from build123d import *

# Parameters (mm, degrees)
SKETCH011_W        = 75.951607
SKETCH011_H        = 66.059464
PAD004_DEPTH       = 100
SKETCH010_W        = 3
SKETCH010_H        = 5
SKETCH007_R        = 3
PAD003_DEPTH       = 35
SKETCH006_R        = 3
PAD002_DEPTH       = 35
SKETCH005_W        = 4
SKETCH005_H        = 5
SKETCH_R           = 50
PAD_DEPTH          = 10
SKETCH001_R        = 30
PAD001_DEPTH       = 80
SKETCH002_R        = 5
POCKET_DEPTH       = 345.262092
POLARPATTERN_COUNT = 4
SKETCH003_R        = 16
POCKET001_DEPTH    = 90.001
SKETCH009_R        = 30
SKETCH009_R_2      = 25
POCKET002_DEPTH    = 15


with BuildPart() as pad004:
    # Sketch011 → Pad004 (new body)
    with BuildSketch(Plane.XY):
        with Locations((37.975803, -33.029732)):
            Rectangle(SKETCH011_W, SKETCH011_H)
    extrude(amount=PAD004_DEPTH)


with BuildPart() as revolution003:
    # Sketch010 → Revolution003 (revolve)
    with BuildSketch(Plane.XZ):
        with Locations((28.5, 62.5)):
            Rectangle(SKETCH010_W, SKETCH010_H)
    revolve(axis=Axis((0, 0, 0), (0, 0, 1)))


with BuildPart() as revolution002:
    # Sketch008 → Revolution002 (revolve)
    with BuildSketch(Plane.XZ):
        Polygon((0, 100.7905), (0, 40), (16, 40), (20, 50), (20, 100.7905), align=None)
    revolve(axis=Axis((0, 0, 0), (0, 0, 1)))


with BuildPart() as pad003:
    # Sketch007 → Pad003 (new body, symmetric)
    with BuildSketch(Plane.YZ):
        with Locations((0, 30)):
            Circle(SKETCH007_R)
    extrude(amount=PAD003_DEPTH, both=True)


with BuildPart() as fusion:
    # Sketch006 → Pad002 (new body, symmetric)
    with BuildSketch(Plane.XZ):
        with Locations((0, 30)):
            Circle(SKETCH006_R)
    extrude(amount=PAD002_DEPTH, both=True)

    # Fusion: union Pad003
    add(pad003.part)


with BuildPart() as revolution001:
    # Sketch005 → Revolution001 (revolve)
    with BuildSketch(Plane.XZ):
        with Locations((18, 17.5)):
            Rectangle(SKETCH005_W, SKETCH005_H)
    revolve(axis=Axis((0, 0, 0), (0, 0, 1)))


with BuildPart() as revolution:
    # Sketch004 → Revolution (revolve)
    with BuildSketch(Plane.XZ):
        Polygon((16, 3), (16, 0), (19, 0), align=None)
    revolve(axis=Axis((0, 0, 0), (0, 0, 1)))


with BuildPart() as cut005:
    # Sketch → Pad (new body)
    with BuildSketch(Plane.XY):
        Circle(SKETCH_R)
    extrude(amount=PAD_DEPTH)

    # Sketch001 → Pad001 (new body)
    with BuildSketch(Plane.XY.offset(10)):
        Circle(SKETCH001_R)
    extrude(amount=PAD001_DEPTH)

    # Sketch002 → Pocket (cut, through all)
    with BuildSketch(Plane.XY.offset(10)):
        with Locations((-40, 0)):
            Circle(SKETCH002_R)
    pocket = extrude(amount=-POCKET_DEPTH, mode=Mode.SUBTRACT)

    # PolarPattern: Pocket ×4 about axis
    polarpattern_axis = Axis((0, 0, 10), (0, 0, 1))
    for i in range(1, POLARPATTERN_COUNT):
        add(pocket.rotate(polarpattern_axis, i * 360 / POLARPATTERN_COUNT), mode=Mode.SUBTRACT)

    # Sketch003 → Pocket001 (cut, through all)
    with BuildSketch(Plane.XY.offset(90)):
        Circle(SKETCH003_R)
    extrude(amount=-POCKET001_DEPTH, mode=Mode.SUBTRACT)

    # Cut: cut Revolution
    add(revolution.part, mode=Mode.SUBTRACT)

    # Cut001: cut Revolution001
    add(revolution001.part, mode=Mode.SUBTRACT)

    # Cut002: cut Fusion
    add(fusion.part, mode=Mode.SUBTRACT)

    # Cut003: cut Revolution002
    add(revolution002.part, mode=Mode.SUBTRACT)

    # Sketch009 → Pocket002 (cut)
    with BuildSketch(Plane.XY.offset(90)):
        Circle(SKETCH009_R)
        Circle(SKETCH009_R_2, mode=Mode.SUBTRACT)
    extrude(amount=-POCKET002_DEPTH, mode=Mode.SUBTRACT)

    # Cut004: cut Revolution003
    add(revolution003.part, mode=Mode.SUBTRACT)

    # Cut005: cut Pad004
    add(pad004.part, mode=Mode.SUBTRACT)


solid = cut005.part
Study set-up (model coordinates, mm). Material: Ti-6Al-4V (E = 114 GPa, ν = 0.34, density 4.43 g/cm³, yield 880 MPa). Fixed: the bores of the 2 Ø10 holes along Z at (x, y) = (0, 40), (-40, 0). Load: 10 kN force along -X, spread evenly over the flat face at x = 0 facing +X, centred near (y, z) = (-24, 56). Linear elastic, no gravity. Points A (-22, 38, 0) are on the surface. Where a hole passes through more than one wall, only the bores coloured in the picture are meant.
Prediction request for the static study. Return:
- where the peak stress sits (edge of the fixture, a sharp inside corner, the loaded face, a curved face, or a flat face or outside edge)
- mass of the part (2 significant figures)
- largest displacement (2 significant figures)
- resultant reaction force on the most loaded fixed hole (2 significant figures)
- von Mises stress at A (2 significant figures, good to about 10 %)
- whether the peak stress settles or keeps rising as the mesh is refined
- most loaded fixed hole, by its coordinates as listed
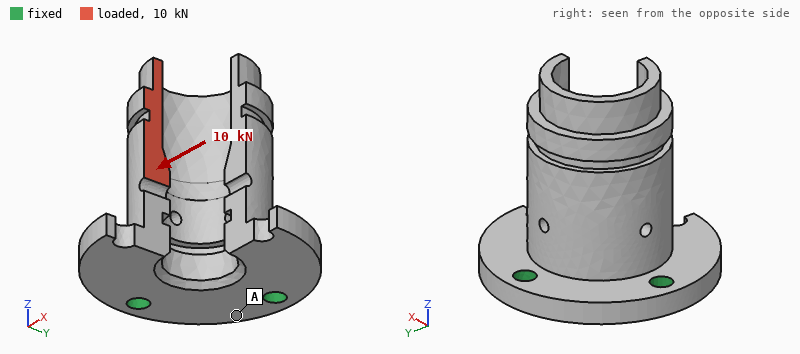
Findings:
edge of the fixture
630 g
0.98 mm
12 kN
43 MPa
keeps rising
(-40, 0)
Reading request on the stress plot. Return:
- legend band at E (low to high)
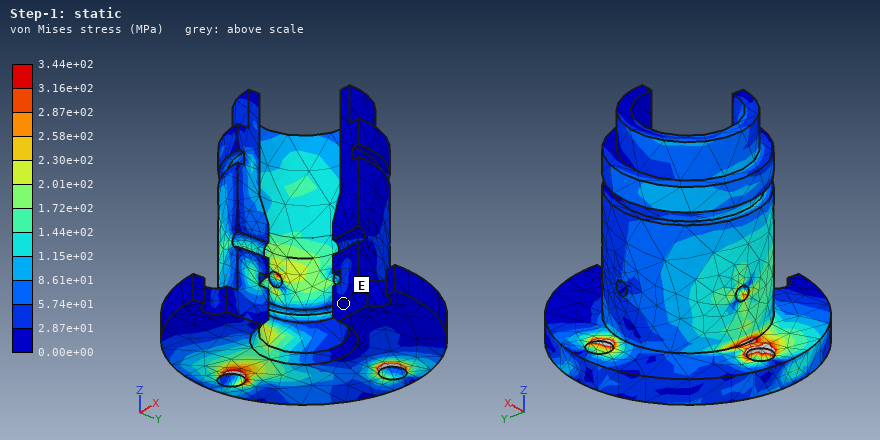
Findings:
0.00e+00 to 2.87e+01 MPa
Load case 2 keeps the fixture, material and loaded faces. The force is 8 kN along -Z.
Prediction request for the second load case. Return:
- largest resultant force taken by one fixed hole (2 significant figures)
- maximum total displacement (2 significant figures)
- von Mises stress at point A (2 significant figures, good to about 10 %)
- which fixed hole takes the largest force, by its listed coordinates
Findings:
7.0 kN
0.59 mm
45 MPa
(-40, 0)
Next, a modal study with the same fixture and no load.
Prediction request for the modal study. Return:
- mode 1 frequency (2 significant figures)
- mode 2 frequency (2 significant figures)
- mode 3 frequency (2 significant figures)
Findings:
1300 Hz
2400 Hz
3200 Hz
